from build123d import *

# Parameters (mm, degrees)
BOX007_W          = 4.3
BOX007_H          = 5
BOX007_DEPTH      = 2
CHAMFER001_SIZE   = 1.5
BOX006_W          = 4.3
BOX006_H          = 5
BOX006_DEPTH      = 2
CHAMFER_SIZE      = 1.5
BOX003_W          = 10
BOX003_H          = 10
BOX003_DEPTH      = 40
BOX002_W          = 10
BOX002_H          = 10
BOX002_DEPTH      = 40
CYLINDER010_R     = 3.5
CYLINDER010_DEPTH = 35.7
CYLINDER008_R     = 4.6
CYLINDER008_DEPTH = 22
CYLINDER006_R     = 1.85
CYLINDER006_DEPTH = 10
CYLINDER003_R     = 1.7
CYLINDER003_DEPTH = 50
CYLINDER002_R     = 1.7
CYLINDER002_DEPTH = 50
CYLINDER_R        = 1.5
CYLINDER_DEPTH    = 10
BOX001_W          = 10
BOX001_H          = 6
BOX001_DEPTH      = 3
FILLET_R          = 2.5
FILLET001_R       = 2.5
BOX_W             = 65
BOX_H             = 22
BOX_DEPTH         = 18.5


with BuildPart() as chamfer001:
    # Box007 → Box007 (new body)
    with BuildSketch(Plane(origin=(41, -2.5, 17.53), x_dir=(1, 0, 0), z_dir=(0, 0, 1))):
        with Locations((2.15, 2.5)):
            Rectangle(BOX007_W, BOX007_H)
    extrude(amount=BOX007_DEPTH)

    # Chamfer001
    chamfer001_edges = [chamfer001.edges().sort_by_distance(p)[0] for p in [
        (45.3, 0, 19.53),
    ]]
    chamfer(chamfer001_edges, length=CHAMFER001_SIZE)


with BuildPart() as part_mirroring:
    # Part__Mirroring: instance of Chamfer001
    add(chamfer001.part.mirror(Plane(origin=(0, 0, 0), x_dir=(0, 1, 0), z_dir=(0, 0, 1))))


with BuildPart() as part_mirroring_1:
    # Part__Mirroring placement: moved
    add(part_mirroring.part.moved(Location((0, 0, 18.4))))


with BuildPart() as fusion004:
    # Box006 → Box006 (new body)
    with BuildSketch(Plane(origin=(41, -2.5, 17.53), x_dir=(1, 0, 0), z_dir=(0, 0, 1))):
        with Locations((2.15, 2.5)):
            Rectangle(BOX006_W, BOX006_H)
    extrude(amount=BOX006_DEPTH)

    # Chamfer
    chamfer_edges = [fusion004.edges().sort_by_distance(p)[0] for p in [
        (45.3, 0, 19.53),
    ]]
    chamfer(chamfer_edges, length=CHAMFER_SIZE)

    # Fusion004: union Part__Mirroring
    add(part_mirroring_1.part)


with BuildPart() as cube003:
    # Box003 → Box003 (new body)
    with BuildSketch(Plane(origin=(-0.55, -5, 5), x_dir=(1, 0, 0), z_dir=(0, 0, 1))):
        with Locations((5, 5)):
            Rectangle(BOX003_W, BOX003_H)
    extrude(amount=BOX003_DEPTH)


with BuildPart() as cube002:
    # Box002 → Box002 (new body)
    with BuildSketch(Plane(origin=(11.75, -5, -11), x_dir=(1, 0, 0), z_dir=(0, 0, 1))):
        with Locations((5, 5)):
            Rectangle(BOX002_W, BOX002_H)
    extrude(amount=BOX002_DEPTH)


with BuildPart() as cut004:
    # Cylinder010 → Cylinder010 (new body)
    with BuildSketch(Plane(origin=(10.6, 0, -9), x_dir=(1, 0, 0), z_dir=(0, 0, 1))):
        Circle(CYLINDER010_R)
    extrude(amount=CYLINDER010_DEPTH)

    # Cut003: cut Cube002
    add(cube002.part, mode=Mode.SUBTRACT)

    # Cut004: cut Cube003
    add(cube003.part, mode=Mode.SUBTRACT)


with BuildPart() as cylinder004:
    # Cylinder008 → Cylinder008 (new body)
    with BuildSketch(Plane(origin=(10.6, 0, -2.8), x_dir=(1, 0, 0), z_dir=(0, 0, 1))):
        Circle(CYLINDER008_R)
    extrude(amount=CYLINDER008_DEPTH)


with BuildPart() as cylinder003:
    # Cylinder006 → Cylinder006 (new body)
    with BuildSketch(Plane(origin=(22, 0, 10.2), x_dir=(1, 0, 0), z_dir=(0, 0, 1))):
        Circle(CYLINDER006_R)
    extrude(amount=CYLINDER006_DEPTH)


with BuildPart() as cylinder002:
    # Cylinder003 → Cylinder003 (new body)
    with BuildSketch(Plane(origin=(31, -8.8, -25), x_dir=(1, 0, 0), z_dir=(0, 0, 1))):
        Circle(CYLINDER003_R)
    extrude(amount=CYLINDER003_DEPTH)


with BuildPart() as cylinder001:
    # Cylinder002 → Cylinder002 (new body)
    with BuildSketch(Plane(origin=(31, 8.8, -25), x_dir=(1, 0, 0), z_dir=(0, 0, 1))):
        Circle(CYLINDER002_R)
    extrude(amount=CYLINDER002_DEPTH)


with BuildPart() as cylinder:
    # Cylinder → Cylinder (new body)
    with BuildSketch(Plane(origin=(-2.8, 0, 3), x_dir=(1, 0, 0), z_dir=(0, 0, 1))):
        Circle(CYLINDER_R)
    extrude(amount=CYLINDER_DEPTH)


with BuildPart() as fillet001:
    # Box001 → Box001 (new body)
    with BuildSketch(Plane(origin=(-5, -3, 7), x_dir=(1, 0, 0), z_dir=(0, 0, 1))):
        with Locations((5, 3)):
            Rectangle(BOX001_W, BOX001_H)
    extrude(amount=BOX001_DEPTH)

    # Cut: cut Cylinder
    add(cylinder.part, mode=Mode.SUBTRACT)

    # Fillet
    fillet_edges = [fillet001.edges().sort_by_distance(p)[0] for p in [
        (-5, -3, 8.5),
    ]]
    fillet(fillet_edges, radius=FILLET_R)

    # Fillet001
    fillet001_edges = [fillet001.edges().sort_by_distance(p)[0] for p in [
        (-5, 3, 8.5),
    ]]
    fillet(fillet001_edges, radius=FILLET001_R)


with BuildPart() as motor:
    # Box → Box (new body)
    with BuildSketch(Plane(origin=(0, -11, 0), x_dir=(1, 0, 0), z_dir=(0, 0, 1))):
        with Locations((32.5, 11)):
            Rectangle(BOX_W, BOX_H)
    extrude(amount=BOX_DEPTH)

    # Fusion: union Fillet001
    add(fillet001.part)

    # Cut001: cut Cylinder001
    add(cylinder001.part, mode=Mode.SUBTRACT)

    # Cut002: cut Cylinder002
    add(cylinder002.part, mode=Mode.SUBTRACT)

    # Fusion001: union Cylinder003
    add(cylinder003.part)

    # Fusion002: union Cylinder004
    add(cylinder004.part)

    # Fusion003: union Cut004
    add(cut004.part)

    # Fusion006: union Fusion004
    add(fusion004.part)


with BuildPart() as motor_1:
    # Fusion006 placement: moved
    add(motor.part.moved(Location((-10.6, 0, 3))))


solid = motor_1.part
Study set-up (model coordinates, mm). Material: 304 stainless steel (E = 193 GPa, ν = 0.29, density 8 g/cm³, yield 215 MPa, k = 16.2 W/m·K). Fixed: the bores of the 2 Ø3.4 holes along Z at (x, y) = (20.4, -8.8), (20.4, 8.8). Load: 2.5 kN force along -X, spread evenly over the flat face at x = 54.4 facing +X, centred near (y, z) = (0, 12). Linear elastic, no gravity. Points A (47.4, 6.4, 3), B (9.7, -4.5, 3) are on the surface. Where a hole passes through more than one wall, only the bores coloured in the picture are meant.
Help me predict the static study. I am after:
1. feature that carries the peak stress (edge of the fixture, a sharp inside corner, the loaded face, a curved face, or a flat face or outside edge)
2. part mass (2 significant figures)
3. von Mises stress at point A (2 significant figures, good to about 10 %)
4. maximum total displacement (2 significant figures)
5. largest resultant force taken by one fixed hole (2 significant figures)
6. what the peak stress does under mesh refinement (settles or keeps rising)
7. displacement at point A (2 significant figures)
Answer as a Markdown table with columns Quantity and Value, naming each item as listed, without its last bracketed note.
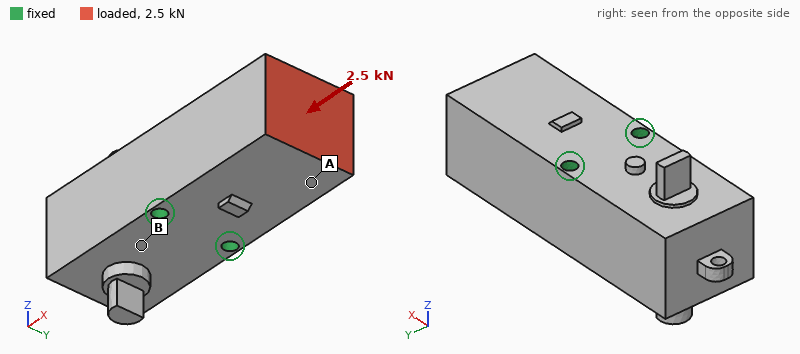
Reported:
| Quantity | Value |
|---|---|
| feature that carries the peak stress | edge of the fixture |
| part mass | 210 g |
| von Mises stress at point A | 6.1 MPa |
| maximum total displacement | 1.1 µm |
| largest resultant force taken by one fixed hole | 1.3 kN |
| what the peak stress does under mesh refinement | keeps rising |
| displacement at point A | 0.90 µm |
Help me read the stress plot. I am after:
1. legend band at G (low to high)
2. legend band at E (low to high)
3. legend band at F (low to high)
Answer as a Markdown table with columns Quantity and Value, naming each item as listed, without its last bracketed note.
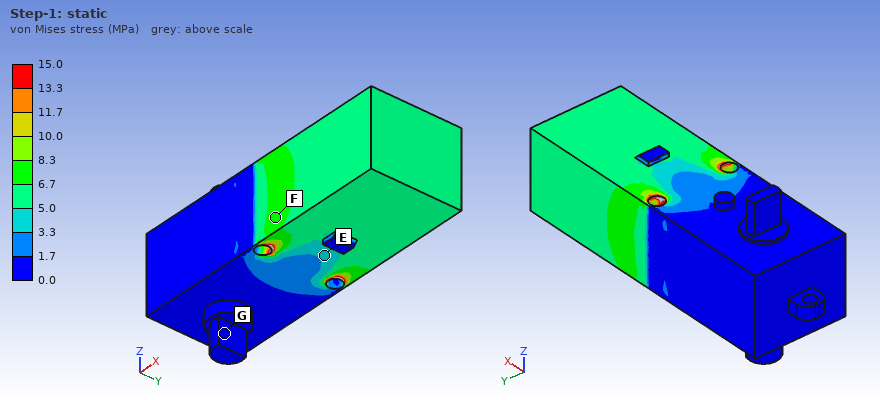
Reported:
| Quantity | Value |
|---|---|
| legend band at G | 0.0 to 1.7 MPa |
| legend band at E | 3.3 to 5.0 MPa |
| legend band at F | 6.7 to 8.3 MPa |
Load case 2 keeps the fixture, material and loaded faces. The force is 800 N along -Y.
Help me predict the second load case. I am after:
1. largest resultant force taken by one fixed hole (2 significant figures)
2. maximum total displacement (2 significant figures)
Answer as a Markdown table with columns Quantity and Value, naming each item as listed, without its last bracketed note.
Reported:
| Quantity | Value |
|---|---|
| largest resultant force taken by one fixed hole | 1.5 kN |
| maximum total displacement | 4.4 µm |
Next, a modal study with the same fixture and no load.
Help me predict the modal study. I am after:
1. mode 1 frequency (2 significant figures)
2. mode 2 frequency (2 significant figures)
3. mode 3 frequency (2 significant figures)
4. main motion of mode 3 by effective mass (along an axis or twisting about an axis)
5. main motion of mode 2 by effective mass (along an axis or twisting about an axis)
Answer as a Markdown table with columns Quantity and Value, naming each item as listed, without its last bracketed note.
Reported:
| Quantity | Value |
|---|---|
| mode 1 frequency | 9800 Hz |
| mode 2 frequency | 12 kHz |
| mode 3 frequency | 13 kHz |
| main motion of mode 3 by effective mass | along Y |
| main motion of mode 2 by effective mass | along Z |
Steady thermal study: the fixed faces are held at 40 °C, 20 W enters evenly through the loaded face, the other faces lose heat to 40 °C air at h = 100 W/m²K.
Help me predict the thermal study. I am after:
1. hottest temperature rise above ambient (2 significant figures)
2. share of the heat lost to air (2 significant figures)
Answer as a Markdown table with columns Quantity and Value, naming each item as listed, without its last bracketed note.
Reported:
| Quantity | Value |
|---|---|
| hottest temperature rise above ambient | 74 K |
| share of the heat lost to air | 46 % |
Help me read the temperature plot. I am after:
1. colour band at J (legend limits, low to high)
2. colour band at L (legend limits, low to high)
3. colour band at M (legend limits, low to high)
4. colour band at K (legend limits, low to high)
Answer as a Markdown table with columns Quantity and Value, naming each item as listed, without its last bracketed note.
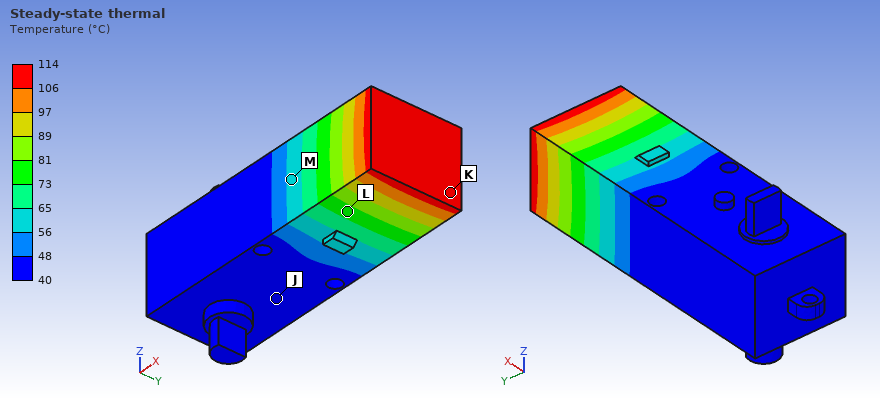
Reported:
| Quantity | Value |
|---|---|
| colour band at J | 40 to 48 °C |
| colour band at L | 73 to 81 °C |
| colour band at M | 56 to 65 °C |
| colour band at K | 106 to 114 °C |
